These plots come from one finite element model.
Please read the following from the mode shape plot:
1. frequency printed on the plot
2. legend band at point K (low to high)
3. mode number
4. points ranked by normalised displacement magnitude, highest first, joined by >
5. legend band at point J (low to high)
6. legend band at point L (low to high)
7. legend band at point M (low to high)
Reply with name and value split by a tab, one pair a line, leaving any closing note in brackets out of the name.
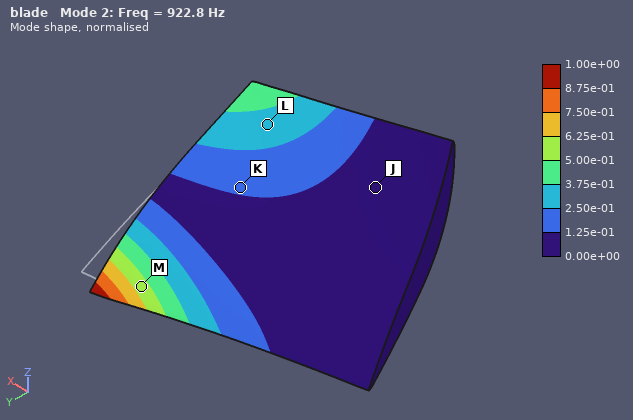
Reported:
frequency printed on the plot	922.8 Hz
legend band at point K	1.25e-01 to 2.50e-01
mode number	2
points ranked by normalised displacement magnitude, highest first, joined by >	M > L > K > J
legend band at point J	0.00e+00 to 1.25e-01
legend band at point L	2.50e-01 to 3.75e-01
legend band at point M	5.00e-01 to 6.25e-01
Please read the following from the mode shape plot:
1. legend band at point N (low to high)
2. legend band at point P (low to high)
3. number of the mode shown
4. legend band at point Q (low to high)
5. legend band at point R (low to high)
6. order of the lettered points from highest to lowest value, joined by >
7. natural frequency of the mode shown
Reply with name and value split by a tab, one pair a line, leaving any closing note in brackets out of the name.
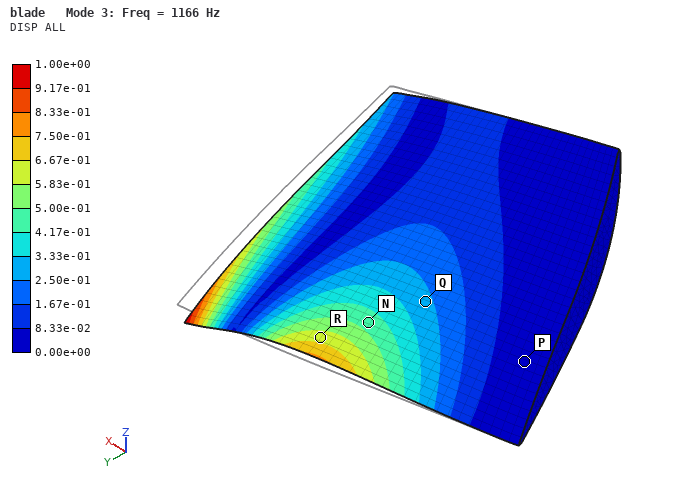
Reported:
legend band at point N	4.17e-01 to 5.00e-01
legend band at point P	0.00e+00 to 8.33e-02
number of the mode shown	3
legend band at point Q	2.50e-01 to 3.33e-01
legend band at point R	5.83e-01 to 6.67e-01
order of the lettered points from highest to lowest value, joined by >	R > N > Q > P
natural frequency of the mode shown	1166 Hz
